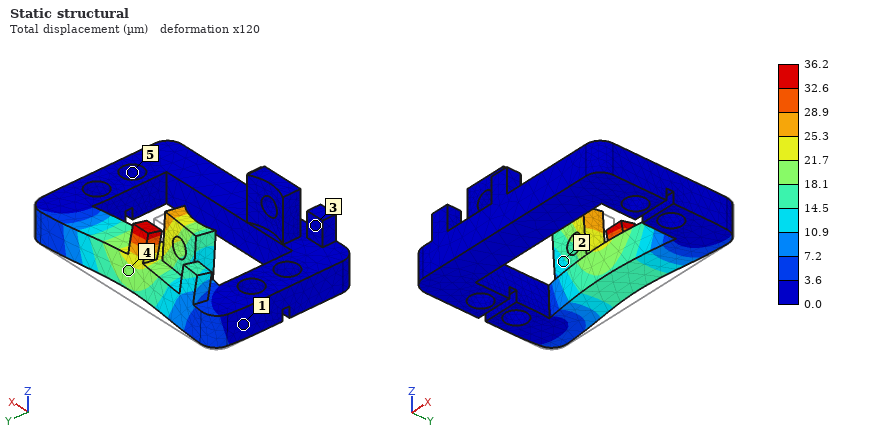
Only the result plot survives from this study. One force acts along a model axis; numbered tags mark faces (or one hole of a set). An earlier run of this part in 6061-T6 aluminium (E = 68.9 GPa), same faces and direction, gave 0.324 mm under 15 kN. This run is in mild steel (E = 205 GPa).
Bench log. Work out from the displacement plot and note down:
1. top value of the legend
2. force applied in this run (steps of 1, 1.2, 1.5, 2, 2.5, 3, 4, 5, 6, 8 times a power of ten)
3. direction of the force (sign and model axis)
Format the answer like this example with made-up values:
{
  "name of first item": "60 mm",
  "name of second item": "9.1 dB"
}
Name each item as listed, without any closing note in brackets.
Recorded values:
{
  "top value of the legend": "36.2 µm",
  "force applied in this run": "5 kN",
  "direction of the force": "-Y"
}
